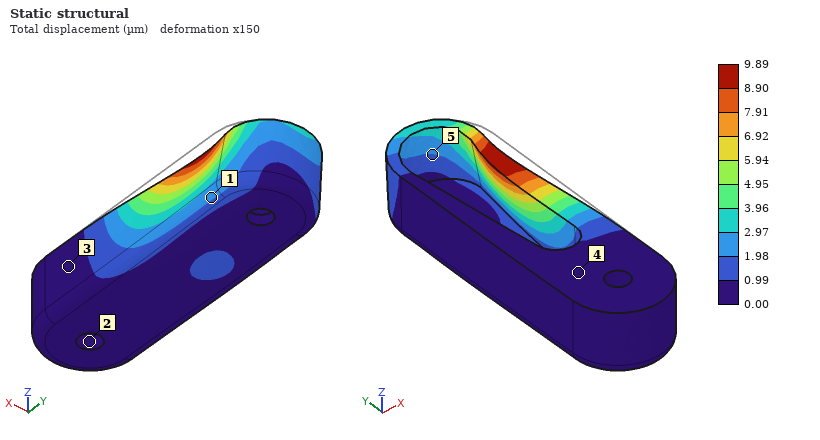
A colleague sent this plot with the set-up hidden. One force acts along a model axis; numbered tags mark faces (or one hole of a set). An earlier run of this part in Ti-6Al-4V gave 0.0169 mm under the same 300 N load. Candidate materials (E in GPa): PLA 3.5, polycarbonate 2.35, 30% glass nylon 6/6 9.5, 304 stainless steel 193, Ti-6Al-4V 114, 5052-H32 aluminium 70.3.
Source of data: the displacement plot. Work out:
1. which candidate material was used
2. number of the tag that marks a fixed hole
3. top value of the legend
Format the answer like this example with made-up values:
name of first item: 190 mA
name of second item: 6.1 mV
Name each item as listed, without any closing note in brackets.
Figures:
which candidate material was used: 304 stainless steel
number of the tag that marks a fixed hole: 2
top value of the legend: 9.89 µm
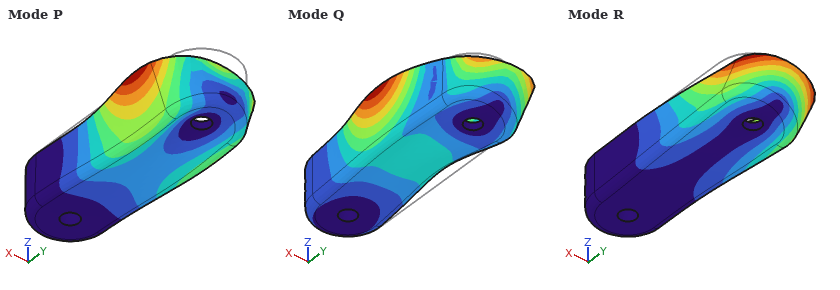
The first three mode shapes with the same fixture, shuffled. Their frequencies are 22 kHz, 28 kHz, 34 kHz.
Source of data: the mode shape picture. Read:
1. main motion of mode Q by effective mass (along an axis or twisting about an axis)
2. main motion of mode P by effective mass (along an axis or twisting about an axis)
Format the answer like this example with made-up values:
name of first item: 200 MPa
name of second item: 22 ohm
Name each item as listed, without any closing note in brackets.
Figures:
main motion of mode Q by effective mass: along X
main motion of mode P by effective mass: along Z
